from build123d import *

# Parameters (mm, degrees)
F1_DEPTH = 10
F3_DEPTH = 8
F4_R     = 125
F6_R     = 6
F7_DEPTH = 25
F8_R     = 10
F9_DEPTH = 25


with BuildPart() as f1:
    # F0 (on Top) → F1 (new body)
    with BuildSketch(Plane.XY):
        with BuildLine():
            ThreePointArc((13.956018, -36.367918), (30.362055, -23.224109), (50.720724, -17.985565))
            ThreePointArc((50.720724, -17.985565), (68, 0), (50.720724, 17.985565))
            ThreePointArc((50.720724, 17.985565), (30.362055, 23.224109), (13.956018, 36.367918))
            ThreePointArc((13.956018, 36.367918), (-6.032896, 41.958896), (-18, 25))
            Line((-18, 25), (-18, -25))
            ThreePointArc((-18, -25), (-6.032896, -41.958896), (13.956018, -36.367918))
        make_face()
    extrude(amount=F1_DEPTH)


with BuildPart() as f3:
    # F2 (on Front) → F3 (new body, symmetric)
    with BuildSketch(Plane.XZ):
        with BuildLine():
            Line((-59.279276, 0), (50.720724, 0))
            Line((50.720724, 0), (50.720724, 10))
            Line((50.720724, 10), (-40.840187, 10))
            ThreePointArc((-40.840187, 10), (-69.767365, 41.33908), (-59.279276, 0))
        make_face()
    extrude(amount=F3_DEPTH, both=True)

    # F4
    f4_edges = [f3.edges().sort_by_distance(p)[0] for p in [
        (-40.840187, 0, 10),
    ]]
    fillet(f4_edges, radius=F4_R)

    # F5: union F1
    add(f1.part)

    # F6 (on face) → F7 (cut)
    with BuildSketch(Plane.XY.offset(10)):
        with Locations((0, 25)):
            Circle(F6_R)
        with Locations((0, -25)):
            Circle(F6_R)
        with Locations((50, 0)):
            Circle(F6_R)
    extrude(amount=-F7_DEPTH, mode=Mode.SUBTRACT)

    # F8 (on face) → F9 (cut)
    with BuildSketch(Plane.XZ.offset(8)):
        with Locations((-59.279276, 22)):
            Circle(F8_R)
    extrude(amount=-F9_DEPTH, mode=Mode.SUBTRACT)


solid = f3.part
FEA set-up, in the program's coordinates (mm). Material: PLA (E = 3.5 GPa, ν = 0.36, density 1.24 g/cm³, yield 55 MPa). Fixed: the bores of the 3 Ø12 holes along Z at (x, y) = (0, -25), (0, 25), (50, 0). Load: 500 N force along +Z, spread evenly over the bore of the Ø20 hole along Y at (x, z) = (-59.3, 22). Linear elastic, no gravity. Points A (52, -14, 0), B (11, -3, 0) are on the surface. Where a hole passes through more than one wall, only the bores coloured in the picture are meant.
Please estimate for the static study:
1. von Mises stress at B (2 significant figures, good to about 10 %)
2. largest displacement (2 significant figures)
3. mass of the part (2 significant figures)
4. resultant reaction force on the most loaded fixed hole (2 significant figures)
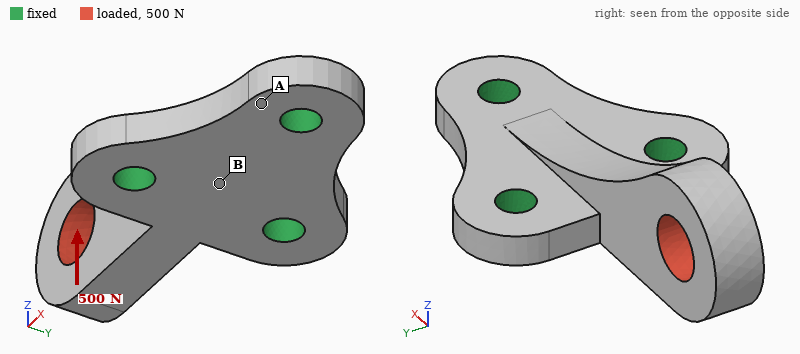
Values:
7.4 MPa
2.1 mm
96 g
500 N
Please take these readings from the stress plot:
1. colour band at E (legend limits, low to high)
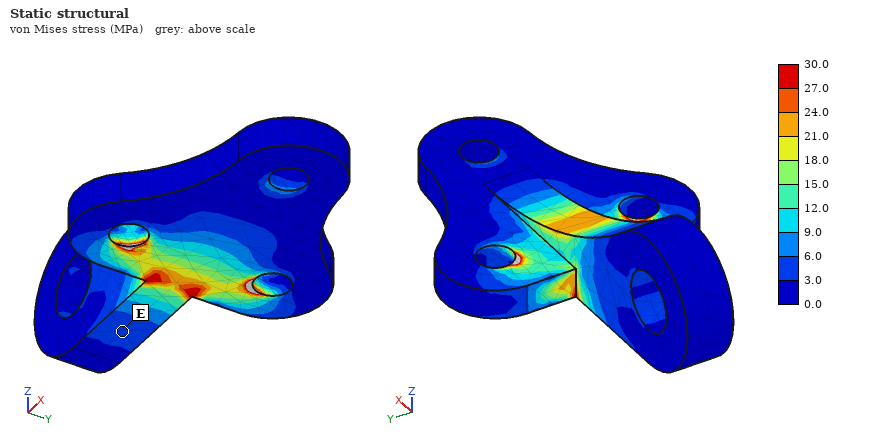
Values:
3.0 to 6.0 MPa
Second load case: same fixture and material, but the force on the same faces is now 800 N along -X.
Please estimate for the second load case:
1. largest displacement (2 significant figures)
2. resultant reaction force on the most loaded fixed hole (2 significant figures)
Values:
0.96 mm
290 N
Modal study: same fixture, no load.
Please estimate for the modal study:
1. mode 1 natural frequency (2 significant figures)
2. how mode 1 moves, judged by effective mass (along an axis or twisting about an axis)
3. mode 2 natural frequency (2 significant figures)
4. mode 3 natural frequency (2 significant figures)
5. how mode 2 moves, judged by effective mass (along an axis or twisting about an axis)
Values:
530 Hz
along Z
690 Hz
1800 Hz
along Y
